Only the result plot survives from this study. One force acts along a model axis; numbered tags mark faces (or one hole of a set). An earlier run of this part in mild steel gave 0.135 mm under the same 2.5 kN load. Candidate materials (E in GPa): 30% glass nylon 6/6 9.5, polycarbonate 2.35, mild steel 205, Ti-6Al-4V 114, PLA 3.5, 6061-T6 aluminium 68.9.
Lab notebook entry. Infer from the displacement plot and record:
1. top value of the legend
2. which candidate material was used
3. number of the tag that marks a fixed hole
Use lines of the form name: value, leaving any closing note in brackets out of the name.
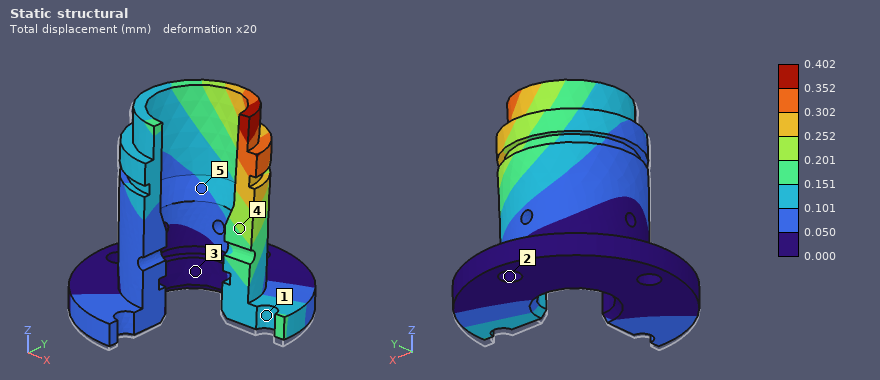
top value of the legend: 0.402 mm
which candidate material was used: 6061-T6 aluminium
number of the tag that marks a fixed hole: 2
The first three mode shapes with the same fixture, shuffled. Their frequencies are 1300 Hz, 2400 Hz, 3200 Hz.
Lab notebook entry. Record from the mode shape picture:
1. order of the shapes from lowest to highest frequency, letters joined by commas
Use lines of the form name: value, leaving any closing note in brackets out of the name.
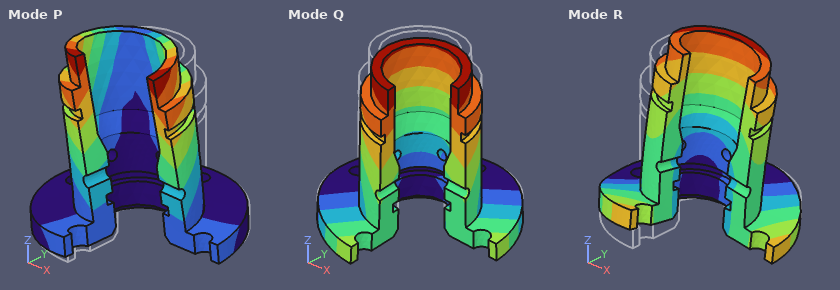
order of the shapes from lowest to highest frequency, letters joined by commas: Q, P, R
